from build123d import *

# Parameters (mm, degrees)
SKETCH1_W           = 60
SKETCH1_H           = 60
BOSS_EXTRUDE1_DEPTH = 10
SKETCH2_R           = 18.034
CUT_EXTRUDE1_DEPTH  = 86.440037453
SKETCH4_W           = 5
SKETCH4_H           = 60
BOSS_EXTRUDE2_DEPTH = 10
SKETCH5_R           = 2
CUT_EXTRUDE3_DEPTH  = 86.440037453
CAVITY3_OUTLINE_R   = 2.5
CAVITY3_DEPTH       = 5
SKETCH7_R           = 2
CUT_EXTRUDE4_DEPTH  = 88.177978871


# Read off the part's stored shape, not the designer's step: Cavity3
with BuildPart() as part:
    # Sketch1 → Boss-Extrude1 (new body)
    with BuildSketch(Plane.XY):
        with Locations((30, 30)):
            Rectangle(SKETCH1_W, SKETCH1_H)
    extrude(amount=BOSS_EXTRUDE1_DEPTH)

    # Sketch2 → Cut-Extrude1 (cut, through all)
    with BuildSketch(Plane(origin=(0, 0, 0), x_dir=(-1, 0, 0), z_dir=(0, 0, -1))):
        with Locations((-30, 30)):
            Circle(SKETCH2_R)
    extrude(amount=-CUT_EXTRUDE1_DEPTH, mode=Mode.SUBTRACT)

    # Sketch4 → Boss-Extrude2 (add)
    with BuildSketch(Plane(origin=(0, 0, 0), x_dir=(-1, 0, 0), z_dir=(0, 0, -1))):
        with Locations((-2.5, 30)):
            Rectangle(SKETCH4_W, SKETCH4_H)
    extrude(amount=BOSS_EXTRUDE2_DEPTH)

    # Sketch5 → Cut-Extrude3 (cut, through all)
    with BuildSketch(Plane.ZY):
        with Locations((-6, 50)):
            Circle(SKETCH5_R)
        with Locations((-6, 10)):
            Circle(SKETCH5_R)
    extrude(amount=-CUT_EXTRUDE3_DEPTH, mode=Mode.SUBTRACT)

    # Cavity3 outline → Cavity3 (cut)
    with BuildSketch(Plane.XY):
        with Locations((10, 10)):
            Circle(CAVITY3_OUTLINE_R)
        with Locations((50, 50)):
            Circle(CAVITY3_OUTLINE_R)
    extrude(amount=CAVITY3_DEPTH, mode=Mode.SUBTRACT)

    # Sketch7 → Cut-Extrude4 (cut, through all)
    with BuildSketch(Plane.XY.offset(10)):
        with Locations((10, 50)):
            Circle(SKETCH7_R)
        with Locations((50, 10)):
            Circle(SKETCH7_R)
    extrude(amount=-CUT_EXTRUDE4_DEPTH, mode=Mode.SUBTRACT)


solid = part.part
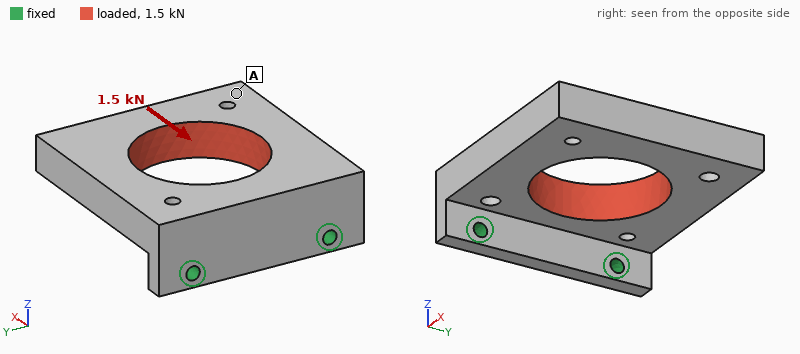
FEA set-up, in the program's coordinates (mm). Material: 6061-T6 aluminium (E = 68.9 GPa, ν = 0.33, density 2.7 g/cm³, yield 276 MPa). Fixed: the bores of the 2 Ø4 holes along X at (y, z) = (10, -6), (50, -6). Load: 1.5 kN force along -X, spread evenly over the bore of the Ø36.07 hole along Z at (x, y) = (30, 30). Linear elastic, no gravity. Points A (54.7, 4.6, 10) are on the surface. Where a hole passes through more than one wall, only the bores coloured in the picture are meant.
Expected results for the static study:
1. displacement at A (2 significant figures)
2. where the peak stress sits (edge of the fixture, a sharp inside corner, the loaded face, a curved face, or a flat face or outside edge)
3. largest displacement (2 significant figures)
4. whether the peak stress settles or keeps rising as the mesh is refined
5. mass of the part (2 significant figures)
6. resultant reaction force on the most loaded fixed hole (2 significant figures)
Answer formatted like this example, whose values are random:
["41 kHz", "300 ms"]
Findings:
["0.17 mm", "edge of the fixture", "0.18 mm", "keeps rising", "76 g", "750 N"]
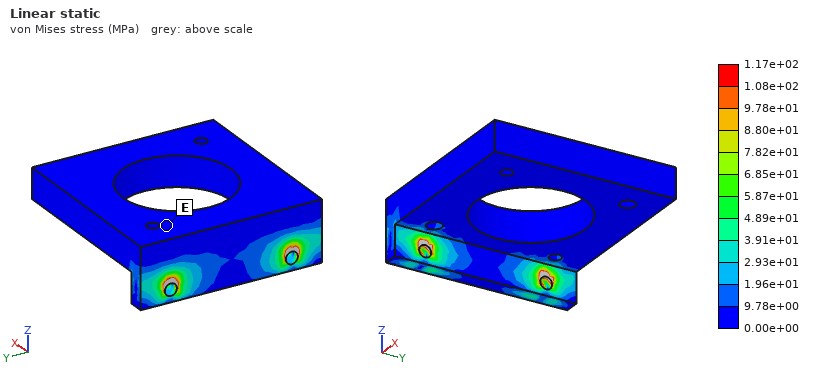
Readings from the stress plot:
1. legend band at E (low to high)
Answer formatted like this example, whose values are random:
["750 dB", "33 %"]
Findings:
["0.00e+00 to 9.78e+00 MPa"]
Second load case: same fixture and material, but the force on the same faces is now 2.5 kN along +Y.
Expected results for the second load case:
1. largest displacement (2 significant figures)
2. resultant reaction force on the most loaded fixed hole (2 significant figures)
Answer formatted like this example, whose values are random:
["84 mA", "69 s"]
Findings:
["0.12 mm", "2.1 kN"]
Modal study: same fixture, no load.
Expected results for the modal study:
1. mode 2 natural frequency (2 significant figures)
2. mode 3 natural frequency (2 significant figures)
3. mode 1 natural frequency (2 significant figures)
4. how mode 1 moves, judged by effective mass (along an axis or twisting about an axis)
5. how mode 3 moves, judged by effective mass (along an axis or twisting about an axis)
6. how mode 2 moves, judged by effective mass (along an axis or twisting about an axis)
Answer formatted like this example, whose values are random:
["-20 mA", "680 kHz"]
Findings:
["2800 Hz", "4000 Hz", "940 Hz", "along Z", "along Y", "along Y"]
